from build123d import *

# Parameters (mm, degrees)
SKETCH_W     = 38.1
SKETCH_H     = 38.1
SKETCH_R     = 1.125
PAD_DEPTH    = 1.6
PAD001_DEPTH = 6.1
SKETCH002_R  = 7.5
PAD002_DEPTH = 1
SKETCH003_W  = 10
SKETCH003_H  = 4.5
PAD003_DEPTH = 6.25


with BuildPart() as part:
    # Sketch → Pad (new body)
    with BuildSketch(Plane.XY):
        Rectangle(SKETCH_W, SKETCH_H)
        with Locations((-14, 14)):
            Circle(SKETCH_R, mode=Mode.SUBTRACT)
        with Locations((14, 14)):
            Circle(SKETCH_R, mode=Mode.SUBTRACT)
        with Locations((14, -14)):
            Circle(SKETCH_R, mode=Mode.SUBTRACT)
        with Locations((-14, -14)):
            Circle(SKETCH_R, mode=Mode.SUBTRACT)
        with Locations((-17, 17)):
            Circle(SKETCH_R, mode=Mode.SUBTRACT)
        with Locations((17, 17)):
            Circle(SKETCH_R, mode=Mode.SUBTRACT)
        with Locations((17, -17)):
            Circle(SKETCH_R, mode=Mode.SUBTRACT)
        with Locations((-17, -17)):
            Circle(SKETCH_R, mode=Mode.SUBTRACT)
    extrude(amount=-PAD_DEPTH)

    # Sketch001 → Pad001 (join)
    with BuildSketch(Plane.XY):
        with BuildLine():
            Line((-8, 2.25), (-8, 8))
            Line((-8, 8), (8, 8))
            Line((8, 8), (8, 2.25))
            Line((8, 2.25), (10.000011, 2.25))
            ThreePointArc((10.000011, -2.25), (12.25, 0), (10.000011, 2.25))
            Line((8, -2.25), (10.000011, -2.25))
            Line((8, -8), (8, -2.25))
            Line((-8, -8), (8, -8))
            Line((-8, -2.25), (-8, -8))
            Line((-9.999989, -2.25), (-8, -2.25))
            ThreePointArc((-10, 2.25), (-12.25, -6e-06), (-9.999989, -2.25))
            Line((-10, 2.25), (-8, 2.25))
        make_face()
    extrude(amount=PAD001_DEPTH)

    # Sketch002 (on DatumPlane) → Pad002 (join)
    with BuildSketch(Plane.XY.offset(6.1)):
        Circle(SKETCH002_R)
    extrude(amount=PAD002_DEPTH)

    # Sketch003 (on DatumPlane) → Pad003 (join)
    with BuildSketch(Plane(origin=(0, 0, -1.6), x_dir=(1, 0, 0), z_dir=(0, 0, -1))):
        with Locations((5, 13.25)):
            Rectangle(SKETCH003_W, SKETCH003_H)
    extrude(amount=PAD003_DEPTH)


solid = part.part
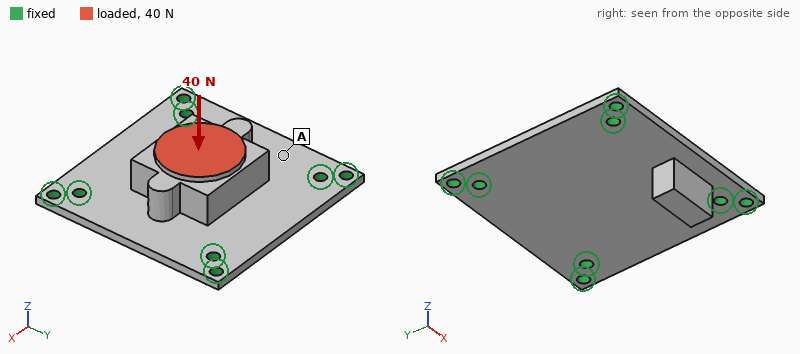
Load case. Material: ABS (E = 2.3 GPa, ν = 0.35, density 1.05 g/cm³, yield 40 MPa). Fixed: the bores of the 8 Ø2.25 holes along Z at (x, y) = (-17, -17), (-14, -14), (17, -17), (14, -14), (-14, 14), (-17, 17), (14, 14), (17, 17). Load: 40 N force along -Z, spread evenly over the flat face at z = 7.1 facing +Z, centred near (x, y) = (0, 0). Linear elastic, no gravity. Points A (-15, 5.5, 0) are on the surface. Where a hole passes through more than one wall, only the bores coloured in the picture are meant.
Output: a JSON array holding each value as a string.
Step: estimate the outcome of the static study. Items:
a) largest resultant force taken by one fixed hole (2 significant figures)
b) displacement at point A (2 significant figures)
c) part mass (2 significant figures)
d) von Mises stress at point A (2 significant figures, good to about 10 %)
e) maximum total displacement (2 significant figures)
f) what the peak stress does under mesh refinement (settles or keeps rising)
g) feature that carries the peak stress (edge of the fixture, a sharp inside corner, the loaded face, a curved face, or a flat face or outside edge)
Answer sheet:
["14 N", "55 µm", "4.7 g", "1.7 MPa", "93 µm", "keeps rising", "edge of the fixture"]
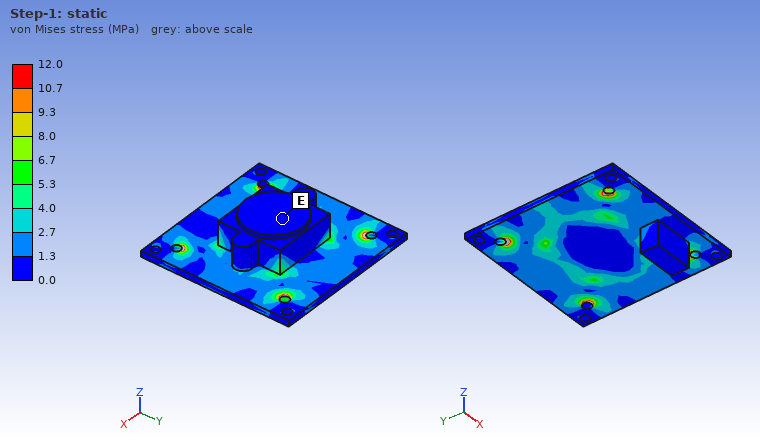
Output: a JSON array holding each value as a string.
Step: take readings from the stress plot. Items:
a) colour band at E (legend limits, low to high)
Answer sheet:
["0.0 to 1.3 MPa"]
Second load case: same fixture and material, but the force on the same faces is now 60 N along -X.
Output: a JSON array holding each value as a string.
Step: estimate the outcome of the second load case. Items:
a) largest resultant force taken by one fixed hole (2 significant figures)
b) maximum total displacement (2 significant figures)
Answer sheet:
["19 N", "0.11 mm"]
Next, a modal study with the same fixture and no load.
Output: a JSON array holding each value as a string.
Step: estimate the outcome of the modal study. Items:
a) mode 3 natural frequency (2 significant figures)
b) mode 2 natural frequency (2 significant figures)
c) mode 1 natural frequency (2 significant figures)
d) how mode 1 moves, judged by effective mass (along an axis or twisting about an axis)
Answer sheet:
["3100 Hz", "2900 Hz", "1900 Hz", "along Z"]
